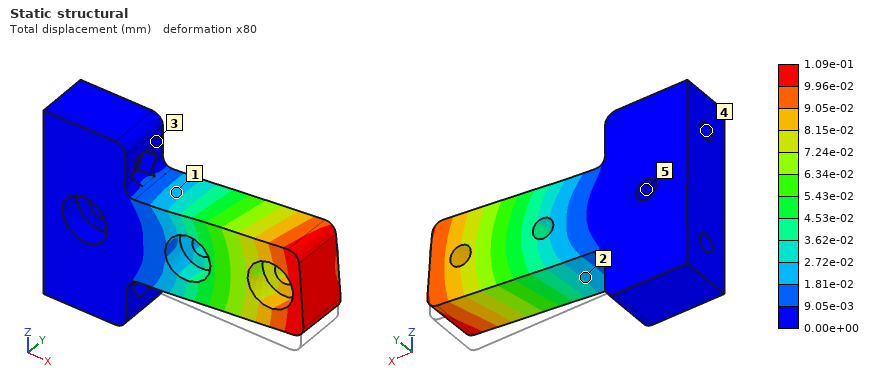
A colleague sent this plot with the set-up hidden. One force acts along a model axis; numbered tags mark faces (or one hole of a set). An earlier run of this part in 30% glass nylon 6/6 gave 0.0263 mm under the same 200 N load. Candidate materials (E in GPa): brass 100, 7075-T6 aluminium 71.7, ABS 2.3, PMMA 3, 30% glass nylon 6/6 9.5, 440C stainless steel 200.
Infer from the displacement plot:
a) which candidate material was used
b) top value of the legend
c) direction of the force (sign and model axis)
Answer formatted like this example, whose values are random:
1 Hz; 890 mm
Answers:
ABS; 1.09e-01 mm; +Z
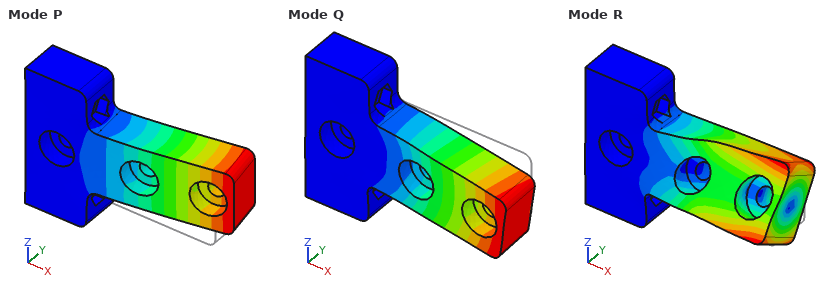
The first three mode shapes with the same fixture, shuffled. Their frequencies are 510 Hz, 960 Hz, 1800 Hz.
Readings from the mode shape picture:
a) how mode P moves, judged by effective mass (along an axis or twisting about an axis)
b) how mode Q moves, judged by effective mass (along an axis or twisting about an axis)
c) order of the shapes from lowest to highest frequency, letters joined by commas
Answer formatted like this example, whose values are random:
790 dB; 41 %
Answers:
along Y; along Z; P, Q, R
